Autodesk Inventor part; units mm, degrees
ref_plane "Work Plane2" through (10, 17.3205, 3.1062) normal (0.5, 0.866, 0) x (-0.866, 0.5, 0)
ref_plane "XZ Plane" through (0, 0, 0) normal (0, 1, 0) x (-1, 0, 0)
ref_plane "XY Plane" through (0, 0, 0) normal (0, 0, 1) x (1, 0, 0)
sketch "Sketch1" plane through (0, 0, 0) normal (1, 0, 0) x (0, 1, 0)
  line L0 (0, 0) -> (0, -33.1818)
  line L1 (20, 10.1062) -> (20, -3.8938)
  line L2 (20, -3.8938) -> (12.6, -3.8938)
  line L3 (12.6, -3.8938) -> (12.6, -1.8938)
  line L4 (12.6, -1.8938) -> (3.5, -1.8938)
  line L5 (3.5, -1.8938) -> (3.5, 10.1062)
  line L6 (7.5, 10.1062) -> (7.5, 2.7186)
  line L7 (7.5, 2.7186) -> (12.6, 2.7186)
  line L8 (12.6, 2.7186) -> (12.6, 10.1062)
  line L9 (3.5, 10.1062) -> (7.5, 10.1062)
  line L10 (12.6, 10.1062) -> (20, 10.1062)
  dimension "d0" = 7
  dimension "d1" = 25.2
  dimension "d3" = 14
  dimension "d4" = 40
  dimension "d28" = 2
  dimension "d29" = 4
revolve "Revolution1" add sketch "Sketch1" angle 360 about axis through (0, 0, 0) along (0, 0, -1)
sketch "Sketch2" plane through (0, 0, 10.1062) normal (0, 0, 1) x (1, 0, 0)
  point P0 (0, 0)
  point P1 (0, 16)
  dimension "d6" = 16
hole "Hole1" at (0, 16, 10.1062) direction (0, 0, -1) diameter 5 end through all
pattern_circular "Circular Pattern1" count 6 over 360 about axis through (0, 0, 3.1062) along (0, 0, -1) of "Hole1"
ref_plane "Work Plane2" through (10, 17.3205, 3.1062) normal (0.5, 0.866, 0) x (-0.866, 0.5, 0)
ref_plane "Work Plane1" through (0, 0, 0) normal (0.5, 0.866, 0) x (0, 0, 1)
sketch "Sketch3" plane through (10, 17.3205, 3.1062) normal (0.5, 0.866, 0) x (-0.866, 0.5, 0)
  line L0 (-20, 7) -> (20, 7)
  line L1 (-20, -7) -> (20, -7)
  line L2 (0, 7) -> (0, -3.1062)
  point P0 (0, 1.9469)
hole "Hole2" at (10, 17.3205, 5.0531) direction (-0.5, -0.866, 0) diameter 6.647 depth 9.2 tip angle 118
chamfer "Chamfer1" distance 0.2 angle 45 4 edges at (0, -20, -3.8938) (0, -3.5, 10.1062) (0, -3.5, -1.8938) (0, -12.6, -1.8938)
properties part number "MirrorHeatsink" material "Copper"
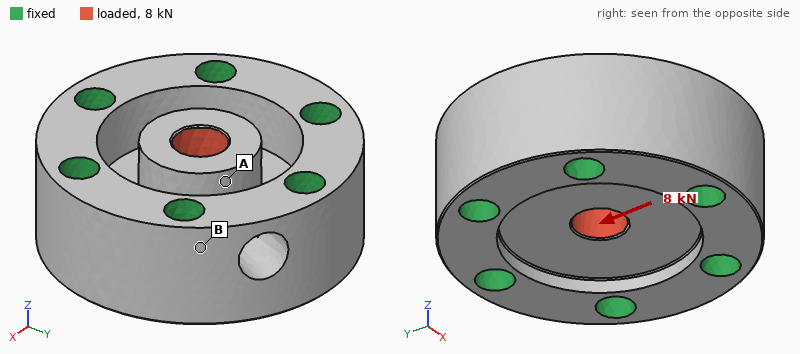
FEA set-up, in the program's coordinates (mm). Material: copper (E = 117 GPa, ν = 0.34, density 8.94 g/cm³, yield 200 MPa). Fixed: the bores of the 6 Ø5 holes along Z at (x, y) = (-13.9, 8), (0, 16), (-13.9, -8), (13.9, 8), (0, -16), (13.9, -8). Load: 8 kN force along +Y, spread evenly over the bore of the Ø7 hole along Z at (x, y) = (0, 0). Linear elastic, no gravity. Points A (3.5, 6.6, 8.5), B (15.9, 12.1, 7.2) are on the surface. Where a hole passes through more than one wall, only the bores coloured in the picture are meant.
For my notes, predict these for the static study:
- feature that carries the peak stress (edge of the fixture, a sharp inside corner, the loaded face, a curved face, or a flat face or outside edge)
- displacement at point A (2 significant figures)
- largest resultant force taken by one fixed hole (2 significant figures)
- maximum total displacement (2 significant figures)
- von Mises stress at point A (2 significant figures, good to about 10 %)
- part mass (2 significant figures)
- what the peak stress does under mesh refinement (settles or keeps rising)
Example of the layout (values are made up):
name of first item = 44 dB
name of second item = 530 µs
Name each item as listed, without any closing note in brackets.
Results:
feature that carries the peak stress = a sharp inside corner
displacement at point A = 13 µm
largest resultant force taken by one fixed hole = 2.3 kN
maximum total displacement = 16 µm
von Mises stress at point A = 27 MPa
part mass = 110 g
what the peak stress does under mesh refinement = keeps rising
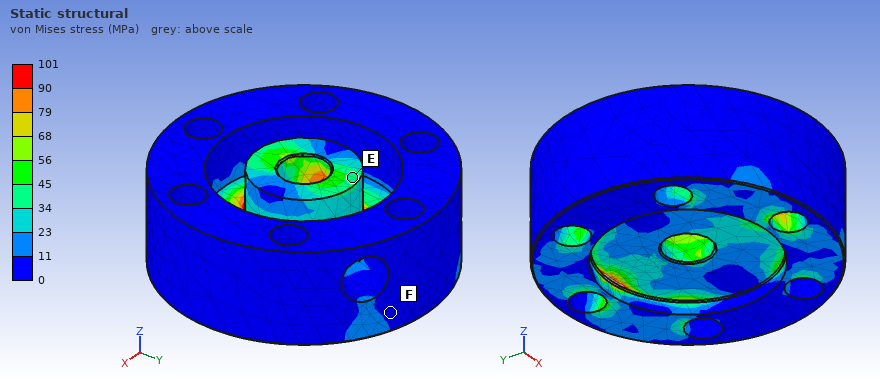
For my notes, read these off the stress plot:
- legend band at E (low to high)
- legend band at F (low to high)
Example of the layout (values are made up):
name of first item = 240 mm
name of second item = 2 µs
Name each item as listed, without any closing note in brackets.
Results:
legend band at E = 34 to 45 MPa
legend band at F = 0 to 11 MPa
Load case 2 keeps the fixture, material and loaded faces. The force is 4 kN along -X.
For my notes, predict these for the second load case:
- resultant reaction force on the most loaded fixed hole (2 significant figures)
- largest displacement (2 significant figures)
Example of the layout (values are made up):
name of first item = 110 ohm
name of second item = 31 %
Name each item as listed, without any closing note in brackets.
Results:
resultant reaction force on the most loaded fixed hole = 1.0 kN
largest displacement = 7.8 µm
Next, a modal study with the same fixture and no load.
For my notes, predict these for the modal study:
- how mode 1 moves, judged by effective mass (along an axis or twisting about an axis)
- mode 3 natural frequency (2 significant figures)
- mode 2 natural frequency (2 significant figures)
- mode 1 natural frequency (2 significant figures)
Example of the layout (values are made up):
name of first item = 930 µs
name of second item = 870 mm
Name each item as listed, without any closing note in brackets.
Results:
how mode 1 moves, judged by effective mass = along Z
mode 3 natural frequency = 33 kHz
mode 2 natural frequency = 33 kHz
mode 1 natural frequency = 31 kHz
